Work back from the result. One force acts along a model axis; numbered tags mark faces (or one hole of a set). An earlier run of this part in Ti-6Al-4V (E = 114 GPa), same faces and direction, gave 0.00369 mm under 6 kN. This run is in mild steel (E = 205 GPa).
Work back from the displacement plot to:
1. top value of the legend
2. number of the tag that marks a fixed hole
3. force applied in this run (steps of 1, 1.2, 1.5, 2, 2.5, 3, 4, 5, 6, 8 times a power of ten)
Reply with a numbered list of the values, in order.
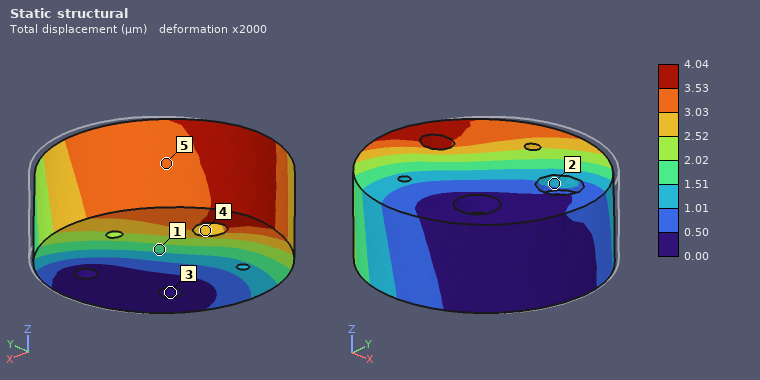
1. 4.04 µm
2. 3
3. 12 kN
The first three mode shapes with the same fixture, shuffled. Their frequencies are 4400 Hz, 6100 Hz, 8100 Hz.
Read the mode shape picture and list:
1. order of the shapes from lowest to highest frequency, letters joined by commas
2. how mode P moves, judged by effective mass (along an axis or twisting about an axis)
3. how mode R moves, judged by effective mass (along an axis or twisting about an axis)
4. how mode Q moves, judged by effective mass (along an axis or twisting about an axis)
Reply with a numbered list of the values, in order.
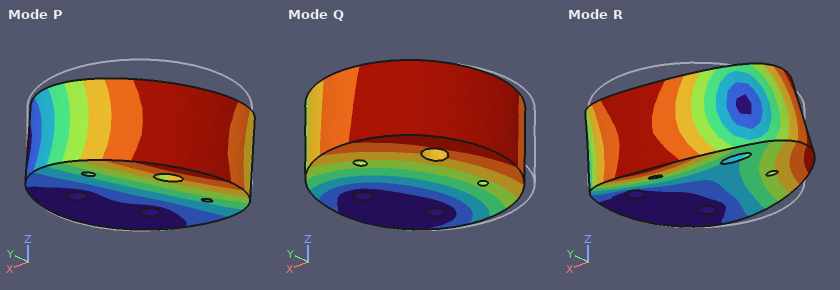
1. P, Q, R
2. along Z
3. twisting about X
4. along Y
